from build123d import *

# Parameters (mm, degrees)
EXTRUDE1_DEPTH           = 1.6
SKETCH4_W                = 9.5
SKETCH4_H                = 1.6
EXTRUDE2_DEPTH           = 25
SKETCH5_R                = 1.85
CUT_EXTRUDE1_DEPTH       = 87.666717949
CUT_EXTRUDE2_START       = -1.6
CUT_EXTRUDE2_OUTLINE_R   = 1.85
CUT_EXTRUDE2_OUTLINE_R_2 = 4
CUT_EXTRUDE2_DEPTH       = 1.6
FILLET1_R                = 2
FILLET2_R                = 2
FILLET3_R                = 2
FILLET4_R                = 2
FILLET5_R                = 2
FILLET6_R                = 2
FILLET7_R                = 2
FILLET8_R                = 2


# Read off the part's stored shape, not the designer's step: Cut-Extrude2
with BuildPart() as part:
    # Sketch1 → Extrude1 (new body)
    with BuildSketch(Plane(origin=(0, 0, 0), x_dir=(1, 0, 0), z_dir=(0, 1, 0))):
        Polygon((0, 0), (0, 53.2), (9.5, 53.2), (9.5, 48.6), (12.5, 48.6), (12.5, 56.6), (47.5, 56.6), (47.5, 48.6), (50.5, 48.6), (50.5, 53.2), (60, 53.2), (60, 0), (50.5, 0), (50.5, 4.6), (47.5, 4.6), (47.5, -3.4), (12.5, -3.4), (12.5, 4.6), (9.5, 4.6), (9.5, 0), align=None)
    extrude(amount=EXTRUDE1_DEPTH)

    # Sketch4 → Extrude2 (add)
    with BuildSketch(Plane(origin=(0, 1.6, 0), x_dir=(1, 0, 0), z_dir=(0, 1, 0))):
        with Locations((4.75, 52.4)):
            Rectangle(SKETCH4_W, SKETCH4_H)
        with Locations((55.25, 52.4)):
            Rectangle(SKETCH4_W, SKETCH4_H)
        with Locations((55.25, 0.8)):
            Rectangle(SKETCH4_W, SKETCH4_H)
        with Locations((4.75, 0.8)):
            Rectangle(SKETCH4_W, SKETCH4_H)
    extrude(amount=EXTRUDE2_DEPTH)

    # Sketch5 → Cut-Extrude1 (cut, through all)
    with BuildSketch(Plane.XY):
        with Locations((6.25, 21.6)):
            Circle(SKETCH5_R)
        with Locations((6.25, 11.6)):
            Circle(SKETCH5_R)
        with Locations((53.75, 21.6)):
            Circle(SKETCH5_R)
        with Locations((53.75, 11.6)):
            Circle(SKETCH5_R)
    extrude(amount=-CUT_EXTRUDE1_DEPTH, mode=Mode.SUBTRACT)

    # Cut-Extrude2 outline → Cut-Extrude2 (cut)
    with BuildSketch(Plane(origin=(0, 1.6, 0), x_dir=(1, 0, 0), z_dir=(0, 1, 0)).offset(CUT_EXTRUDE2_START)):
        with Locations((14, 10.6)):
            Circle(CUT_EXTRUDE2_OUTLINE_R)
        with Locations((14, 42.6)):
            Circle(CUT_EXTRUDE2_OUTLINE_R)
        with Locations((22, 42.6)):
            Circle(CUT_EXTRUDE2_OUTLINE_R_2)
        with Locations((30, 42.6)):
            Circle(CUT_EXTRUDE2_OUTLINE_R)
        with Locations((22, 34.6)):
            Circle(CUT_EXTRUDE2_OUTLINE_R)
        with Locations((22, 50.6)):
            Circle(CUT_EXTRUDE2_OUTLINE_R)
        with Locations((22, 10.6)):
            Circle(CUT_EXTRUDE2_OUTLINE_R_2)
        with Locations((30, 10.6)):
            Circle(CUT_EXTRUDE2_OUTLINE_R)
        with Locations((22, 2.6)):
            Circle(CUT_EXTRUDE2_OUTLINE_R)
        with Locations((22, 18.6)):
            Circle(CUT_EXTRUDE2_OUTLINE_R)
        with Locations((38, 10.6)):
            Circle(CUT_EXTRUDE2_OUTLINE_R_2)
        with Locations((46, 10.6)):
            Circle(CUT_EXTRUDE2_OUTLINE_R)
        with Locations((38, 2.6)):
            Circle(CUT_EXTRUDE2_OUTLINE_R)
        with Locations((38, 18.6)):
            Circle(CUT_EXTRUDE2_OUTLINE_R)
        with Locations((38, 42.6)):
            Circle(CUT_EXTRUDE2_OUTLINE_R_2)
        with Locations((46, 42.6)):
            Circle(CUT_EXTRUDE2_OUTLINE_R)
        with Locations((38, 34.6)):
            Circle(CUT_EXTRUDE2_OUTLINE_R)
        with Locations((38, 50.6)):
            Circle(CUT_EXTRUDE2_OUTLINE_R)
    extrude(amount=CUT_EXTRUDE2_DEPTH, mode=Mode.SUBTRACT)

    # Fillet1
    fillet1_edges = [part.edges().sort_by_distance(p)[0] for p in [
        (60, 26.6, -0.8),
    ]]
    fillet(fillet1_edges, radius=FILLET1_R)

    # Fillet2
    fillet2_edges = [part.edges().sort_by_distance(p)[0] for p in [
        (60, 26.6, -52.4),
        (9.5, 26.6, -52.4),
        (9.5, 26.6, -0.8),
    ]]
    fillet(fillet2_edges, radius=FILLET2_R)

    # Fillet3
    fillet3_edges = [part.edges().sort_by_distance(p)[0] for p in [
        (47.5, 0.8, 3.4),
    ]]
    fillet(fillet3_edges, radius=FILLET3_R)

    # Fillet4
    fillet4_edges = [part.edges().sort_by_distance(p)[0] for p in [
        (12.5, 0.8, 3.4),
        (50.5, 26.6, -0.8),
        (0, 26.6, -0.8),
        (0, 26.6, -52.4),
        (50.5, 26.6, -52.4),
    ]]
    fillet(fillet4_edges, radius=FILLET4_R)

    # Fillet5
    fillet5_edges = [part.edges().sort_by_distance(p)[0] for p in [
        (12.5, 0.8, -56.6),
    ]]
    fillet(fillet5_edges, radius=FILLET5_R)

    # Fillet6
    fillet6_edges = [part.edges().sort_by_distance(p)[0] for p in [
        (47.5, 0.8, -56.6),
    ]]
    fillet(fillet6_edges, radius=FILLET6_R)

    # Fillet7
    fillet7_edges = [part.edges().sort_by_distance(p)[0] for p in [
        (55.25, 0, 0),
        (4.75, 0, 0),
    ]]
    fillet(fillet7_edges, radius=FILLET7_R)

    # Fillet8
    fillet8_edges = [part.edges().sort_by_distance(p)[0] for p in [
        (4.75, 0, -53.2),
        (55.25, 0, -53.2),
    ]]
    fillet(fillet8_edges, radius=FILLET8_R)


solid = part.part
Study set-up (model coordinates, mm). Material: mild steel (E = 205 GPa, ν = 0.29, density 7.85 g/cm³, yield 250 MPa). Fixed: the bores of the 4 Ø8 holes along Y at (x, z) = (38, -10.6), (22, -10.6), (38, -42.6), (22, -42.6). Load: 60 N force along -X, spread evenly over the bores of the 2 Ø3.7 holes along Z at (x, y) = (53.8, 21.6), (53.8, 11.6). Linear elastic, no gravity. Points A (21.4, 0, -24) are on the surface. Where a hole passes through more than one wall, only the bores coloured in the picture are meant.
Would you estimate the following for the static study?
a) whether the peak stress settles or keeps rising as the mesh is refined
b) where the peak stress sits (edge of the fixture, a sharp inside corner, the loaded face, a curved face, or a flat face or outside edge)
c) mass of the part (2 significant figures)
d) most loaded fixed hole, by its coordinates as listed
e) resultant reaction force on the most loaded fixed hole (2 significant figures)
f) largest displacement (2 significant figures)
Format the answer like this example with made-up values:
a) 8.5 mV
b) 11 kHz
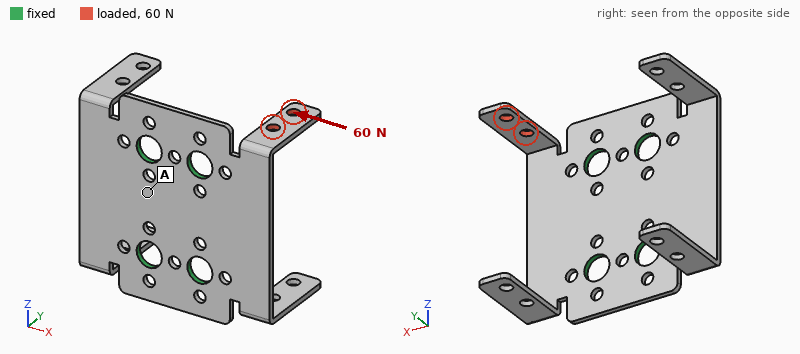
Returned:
a) keeps rising
b) a sharp inside corner
c) 48 g
d) (38, -10.6)
e) 71 N
f) 0.41 mm
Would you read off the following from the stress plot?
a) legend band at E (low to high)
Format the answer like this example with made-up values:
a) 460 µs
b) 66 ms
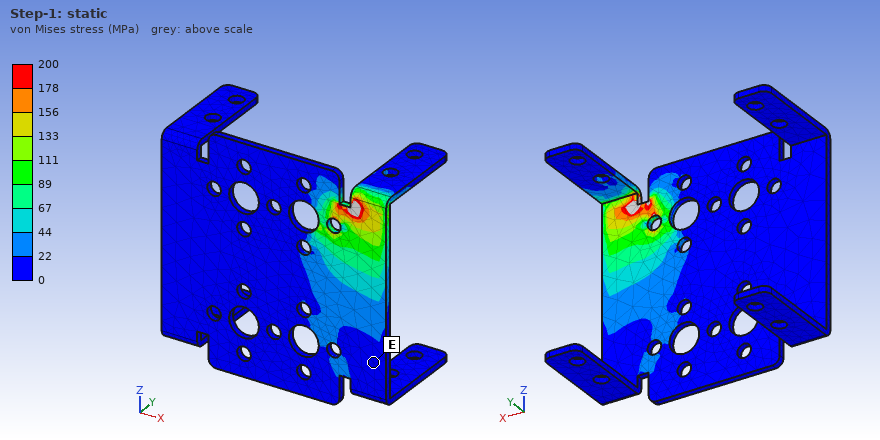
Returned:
a) 0 to 22 MPa
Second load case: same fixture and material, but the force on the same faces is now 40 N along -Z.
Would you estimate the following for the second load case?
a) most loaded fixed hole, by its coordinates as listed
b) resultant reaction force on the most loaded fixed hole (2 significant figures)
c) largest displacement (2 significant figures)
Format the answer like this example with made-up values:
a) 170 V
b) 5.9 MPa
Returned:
a) (38, -10.6)
b) 30 N
c) 0.43 mm
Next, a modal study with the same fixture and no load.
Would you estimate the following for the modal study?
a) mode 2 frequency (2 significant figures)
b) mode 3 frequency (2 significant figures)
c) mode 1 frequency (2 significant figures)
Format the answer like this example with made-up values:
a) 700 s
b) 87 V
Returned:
a) 1200 Hz
b) 1200 Hz
c) 1200 Hz
